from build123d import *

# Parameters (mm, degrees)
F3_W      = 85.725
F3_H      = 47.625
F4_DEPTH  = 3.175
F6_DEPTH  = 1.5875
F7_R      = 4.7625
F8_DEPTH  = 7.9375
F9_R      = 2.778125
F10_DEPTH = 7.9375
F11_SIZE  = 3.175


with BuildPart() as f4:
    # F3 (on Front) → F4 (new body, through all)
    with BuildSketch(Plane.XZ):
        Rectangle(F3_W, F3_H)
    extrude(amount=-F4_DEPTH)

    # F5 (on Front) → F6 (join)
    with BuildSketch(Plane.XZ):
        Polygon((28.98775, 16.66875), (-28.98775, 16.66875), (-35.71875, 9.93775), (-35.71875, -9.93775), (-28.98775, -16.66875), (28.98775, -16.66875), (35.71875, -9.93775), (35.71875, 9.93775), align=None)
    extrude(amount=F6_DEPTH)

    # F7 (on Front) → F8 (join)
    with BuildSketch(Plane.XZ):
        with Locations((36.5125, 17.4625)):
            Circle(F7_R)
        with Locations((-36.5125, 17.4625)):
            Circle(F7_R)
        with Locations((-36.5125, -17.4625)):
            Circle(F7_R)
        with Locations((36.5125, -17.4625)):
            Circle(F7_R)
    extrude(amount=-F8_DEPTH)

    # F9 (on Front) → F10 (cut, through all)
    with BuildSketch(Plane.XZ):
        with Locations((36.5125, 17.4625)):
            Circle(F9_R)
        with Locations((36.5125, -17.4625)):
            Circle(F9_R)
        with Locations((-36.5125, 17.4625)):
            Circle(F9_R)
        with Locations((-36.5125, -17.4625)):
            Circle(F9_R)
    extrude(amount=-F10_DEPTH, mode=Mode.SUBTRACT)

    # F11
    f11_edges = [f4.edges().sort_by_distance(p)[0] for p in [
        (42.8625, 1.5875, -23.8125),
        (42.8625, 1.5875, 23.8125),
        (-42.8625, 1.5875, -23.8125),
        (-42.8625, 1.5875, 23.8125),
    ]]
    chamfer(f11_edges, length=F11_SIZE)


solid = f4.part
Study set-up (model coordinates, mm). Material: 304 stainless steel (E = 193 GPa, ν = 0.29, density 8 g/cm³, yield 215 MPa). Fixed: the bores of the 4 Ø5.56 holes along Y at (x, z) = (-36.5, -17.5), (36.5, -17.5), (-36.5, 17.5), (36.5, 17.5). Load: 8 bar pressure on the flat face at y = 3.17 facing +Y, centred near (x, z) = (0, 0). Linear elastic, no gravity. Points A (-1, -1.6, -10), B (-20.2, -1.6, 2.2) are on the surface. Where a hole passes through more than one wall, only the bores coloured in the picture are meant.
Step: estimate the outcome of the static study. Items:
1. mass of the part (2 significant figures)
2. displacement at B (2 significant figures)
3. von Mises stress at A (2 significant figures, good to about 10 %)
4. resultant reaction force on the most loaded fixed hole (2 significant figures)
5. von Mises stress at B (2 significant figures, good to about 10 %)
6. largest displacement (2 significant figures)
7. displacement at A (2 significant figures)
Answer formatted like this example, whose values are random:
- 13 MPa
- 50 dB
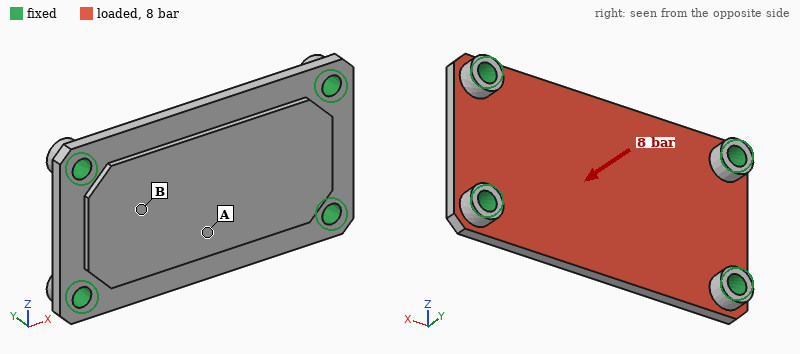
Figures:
- 140 g
- 30 µm
- 70 MPa
- 1.0 kN
- 21 MPa
- 59 µm
- 53 µm
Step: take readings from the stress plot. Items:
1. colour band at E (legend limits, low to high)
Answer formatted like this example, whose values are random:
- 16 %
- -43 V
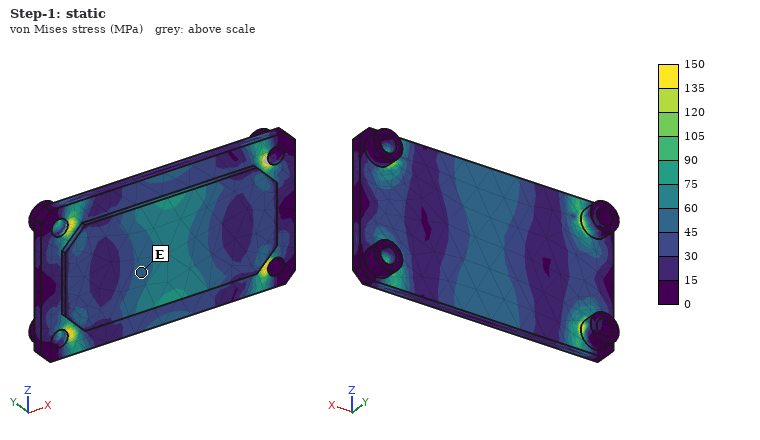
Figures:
- 45 to 60 MPa
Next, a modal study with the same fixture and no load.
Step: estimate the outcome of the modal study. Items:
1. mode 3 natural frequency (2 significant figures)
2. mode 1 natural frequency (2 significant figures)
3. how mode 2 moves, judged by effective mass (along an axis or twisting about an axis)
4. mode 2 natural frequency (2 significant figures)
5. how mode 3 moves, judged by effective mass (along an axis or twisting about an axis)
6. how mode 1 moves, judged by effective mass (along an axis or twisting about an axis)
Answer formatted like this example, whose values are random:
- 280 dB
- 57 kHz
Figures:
- 10 kHz
- 3700 Hz
- twisting about X
- 6000 Hz
- twisting about Z
- along Y
